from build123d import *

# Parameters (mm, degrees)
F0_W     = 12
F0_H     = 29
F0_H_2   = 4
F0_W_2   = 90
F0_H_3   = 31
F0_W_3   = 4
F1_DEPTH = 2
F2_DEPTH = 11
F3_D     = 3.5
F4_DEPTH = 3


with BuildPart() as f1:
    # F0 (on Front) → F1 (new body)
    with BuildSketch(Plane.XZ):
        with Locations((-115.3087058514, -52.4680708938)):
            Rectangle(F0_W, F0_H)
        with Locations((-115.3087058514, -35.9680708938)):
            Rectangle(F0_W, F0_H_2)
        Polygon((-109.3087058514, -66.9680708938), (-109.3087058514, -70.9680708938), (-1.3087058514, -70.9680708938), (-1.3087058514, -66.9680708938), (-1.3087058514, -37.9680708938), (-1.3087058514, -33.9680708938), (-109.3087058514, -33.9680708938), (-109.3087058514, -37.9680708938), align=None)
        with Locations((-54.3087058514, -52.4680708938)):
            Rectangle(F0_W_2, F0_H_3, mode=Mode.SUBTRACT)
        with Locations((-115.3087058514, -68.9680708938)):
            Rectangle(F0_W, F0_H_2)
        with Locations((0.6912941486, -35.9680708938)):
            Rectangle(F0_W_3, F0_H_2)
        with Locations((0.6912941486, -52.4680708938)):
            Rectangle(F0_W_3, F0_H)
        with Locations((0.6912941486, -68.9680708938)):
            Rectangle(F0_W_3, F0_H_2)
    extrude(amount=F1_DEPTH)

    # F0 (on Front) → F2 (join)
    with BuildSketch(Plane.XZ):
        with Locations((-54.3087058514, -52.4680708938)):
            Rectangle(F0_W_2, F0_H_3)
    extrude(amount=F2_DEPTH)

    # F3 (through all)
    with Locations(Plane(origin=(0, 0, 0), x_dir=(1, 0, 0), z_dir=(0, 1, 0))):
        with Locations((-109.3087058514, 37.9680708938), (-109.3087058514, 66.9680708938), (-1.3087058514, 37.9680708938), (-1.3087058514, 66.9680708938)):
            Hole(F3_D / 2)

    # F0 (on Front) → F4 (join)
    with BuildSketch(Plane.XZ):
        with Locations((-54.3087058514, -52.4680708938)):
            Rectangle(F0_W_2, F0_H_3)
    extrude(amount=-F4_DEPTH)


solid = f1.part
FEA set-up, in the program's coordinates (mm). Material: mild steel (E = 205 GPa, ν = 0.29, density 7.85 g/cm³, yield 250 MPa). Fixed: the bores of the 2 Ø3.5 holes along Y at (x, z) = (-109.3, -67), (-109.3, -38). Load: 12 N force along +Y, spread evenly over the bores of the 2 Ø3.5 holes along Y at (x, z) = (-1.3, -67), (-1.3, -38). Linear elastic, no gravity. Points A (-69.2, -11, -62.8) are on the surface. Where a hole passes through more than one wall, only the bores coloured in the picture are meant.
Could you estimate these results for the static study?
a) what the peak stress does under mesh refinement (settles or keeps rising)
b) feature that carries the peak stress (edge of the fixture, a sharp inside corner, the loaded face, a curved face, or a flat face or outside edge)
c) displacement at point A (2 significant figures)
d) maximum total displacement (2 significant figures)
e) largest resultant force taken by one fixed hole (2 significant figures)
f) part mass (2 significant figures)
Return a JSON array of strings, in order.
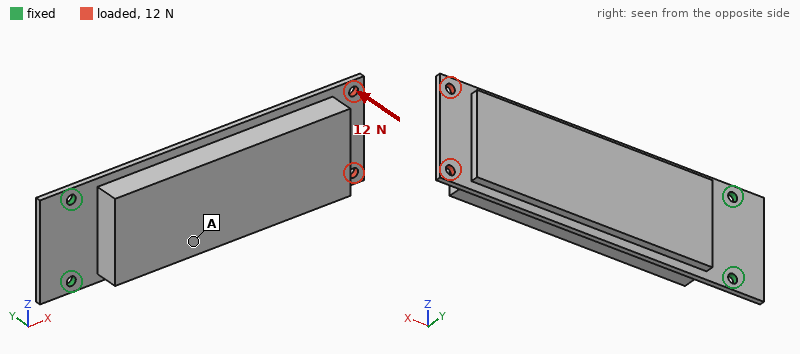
["keeps rising", "edge of the fixture", "0.092 mm", "0.27 mm", "6.1 N", "330 g"]
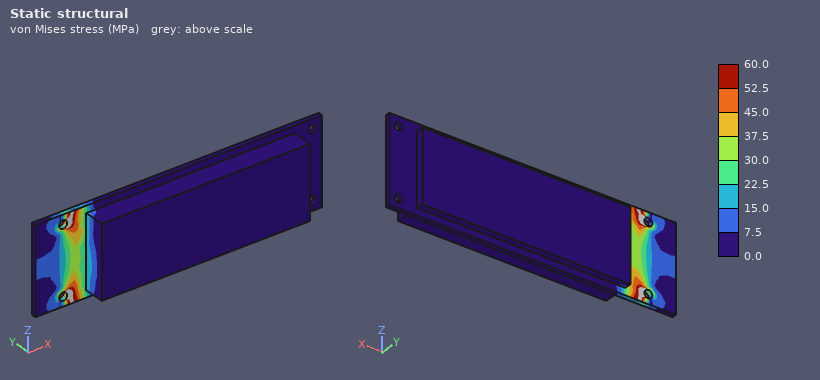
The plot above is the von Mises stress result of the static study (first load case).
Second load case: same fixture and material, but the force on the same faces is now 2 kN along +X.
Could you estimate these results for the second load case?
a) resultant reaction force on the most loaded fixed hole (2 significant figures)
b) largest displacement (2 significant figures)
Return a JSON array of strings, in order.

["1.0 kN", "21 µm"]
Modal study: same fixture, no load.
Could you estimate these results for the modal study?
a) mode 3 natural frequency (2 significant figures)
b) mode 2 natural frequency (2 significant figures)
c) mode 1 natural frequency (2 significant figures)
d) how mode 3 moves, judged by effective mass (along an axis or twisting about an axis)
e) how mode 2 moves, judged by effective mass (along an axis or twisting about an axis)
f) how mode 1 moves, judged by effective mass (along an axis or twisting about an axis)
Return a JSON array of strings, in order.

["2100 Hz", "1500 Hz", "110 Hz", "twisting about X", "along Z", "along Y"]
